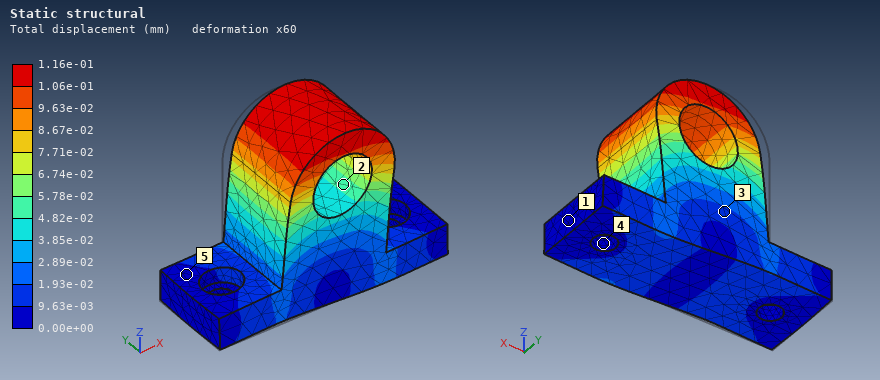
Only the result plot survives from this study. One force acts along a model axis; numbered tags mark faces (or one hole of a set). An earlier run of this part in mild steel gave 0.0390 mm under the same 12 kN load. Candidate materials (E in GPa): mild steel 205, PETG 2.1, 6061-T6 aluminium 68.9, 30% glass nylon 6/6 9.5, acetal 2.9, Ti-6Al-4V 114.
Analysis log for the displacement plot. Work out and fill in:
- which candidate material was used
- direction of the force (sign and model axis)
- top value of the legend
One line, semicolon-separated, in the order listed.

6061-T6 aluminium; +X; 1.16e-01 mm
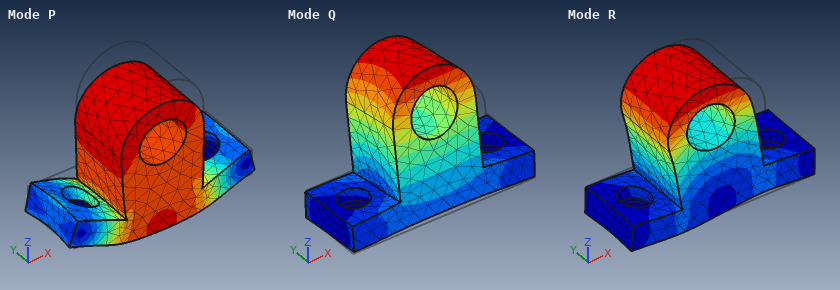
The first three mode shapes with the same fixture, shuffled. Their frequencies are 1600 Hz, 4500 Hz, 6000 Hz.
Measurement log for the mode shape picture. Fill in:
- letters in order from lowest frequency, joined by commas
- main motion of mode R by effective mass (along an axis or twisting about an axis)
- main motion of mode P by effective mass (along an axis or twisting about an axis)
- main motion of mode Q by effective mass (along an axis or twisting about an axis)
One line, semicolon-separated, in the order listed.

Q, R, P; along X; along Z; along Y
